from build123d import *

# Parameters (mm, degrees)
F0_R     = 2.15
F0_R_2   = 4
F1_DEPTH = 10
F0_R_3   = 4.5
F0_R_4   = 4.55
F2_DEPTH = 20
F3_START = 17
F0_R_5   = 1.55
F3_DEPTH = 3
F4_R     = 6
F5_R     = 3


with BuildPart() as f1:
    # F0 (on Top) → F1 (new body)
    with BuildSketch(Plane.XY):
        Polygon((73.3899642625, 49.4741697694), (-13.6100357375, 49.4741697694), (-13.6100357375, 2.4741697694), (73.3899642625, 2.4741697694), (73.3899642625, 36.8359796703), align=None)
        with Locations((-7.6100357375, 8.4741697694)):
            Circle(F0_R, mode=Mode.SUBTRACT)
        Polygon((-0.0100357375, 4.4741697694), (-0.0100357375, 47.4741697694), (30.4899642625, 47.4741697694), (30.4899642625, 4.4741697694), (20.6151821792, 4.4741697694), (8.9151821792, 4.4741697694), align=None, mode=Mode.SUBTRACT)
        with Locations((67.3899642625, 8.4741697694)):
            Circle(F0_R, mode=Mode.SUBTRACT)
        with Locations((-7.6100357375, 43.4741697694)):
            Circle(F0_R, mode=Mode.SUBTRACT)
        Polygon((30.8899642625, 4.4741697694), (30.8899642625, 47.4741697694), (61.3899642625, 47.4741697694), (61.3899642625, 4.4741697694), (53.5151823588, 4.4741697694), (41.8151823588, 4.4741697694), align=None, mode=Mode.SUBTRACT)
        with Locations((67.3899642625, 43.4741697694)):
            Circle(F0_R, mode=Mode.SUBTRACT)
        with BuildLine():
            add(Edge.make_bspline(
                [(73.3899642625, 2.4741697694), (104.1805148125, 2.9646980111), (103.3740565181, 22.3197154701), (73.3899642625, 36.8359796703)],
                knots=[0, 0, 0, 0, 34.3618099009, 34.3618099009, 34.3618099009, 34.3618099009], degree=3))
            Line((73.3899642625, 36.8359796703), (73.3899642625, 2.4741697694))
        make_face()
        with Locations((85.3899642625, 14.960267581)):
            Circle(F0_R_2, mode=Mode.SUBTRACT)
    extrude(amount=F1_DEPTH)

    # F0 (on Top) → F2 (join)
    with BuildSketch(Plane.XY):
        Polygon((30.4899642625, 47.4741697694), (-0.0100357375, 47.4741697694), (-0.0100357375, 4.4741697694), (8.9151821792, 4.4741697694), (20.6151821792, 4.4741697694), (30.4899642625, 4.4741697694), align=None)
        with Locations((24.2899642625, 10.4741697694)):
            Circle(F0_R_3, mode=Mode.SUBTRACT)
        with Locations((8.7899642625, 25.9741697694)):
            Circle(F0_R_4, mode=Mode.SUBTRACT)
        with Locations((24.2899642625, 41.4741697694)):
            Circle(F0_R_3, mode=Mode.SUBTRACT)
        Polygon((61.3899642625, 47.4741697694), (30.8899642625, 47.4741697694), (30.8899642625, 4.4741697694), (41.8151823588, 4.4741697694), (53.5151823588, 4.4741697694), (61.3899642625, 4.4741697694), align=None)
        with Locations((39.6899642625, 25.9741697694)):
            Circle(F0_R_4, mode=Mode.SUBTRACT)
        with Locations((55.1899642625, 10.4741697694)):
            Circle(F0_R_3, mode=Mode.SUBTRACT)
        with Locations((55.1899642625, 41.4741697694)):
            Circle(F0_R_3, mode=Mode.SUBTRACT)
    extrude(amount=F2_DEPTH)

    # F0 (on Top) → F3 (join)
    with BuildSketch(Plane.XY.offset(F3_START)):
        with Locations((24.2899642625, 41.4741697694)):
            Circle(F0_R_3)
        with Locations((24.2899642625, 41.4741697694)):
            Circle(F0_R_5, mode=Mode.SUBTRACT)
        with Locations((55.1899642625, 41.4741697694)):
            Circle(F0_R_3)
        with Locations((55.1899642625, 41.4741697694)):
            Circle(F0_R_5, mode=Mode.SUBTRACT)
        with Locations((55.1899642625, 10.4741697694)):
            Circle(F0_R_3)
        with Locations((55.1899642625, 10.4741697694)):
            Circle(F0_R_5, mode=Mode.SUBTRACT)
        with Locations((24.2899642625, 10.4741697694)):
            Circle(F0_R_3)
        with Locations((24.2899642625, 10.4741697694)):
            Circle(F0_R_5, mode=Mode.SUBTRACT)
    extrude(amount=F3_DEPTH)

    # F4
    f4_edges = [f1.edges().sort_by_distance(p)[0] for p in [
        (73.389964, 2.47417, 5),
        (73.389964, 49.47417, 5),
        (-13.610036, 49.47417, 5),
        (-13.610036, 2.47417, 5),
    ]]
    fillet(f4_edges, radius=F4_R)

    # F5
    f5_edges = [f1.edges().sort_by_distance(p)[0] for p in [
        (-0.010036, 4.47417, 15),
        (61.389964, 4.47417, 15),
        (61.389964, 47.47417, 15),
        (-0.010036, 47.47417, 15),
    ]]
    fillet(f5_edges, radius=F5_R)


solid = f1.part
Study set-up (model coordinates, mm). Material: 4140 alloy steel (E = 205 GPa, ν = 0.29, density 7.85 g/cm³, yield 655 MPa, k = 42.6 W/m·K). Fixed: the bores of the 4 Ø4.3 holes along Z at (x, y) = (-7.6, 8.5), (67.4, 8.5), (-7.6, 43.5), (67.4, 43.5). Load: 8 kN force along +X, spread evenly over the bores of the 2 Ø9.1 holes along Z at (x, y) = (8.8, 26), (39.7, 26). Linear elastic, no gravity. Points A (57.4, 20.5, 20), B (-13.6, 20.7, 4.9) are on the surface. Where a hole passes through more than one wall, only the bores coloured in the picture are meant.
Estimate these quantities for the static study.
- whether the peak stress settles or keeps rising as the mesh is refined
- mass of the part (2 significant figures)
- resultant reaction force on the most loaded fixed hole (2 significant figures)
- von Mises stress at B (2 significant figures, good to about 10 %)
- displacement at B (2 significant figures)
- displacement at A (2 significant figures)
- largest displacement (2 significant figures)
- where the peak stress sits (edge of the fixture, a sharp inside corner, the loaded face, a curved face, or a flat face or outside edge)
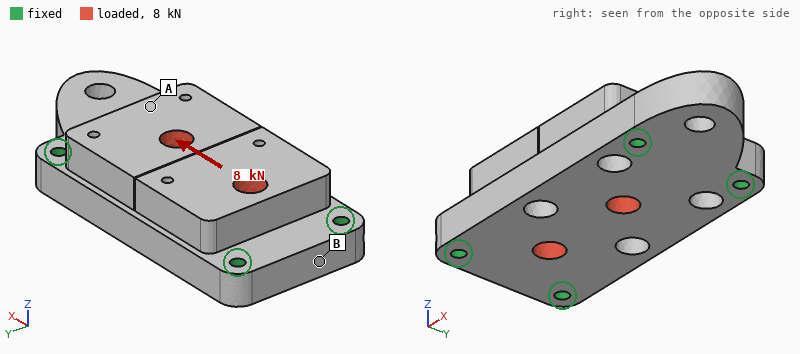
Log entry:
keeps rising
500 g
2.4 kN
8.6 MPa
1.2 µm
1.6 µm
2.7 µm
edge of the fixture
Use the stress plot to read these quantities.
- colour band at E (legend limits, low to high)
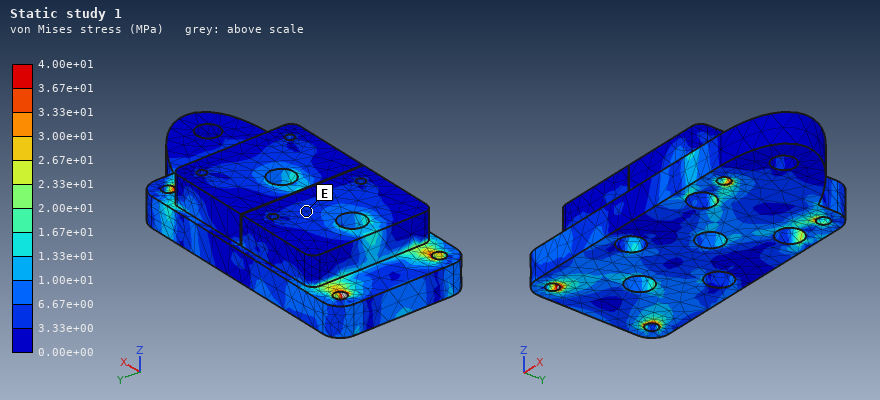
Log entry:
3.33e+00 to 6.67e+00 MPa
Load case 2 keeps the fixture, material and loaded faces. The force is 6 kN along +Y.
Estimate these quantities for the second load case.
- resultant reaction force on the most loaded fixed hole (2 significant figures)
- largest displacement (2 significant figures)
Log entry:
2.2 kN
3.4 µm
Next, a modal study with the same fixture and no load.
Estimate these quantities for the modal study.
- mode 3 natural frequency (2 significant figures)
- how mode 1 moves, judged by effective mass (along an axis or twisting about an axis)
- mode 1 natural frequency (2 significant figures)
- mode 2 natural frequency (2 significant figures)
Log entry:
12 kHz
along Z
6200 Hz
11 kHz
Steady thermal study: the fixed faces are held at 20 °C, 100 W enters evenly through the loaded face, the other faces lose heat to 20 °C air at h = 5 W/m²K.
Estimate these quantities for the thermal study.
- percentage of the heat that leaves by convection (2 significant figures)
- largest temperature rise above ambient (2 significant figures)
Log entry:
3.1 %
72 K
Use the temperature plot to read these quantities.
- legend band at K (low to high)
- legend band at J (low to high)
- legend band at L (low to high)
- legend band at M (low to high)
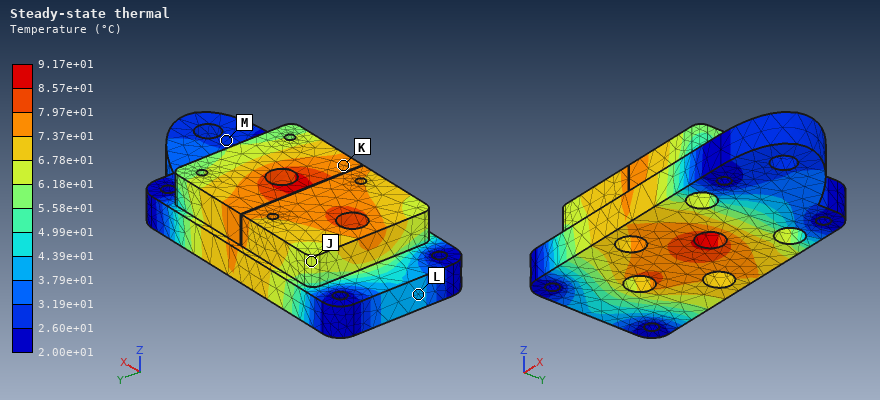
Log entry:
7.37e+01 to 7.97e+01 °C
6.18e+01 to 6.78e+01 °C
3.79e+01 to 4.39e+01 °C
2.60e+01 to 3.19e+01 °C
